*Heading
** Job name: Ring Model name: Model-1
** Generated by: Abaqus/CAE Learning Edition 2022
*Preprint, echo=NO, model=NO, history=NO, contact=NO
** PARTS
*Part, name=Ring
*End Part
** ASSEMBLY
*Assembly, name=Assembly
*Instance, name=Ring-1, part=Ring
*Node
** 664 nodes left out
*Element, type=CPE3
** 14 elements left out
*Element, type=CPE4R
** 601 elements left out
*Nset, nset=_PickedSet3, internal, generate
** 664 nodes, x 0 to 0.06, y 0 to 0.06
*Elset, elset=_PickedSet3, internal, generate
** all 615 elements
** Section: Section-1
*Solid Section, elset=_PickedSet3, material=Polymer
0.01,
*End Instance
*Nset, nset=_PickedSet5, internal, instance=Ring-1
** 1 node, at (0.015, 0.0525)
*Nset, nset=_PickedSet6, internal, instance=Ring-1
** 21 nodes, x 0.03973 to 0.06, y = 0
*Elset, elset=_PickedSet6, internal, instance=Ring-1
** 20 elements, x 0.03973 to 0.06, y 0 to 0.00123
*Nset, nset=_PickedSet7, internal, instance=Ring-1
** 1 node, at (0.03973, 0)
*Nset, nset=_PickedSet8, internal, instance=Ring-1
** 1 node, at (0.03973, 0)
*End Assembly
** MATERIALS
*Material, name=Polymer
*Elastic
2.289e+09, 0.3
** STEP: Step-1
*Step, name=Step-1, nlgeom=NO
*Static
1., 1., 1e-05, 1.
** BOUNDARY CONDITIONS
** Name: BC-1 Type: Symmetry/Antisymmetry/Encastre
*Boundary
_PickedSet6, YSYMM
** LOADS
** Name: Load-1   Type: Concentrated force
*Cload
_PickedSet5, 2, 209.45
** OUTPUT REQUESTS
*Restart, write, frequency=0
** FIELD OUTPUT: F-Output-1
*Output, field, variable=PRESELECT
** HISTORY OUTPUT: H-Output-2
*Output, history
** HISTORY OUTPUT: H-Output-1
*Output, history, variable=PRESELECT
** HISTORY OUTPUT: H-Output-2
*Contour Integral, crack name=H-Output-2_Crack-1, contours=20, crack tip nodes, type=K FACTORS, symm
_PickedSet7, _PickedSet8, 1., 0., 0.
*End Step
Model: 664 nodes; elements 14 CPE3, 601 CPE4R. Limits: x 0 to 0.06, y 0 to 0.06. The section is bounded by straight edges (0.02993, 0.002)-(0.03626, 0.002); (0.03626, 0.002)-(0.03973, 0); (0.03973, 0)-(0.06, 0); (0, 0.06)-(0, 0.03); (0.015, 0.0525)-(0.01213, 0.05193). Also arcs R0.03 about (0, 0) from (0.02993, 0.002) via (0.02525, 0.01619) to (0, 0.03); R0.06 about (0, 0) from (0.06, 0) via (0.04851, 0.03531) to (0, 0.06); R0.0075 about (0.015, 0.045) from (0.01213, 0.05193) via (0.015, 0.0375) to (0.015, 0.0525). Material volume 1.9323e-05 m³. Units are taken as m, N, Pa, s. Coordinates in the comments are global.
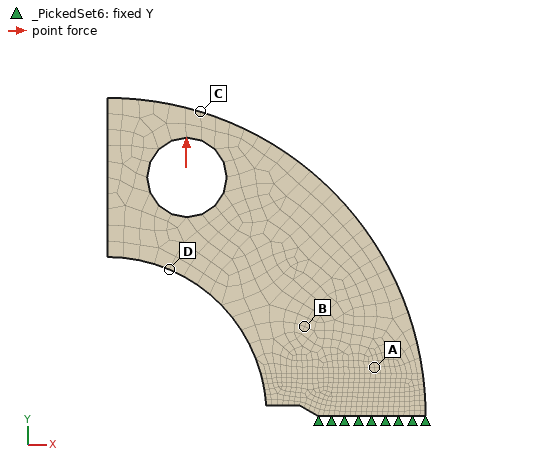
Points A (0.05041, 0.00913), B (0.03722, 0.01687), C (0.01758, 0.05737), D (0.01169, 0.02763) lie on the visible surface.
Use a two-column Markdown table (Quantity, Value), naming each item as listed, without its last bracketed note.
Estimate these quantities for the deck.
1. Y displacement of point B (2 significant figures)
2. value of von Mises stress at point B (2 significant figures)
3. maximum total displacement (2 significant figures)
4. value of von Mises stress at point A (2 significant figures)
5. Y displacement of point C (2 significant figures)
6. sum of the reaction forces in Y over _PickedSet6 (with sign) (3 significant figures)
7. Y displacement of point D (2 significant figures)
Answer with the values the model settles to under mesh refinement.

| Quantity | Value |
|---|---|
| Y displacement of point B | 5.0e-05 m |
| value of von Mises stress at point B | 2.0e+06 Pa |
| maximum total displacement | 4.3e-04 m |
| value of von Mises stress at point A | 2.6e+06 Pa |
| Y displacement of point C | 2.5e-04 m |
| sum of the reaction forces in Y over _PickedSet6 (with sign) | -209 N |
| Y displacement of point D | 2.4e-04 m |
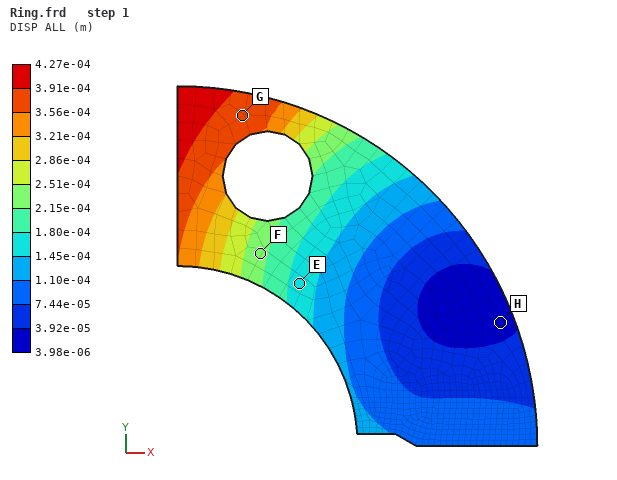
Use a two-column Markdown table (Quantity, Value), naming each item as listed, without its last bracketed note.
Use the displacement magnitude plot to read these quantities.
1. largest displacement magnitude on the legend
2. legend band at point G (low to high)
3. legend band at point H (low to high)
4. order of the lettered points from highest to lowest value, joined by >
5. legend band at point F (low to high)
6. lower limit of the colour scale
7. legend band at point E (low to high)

| Quantity | Value |
|---|---|
| largest displacement magnitude on the legend | 4.27e-04 m |
| legend band at point G | 3.56e-04 to 3.91e-04 m |
| legend band at point H | 3.98e-06 to 3.92e-05 m |
| order of the lettered points from highest to lowest value, joined by > | G > F > E > H |
| legend band at point F | 2.15e-04 to 2.51e-04 m |
| lower limit of the colour scale | 3.98e-06 m |
| legend band at point E | 1.45e-04 to 1.80e-04 m |
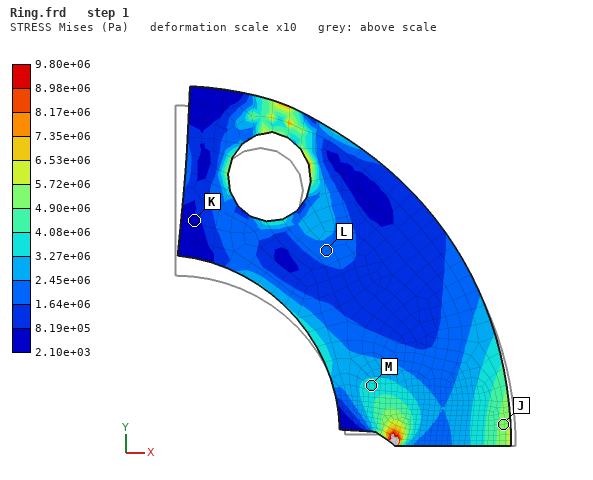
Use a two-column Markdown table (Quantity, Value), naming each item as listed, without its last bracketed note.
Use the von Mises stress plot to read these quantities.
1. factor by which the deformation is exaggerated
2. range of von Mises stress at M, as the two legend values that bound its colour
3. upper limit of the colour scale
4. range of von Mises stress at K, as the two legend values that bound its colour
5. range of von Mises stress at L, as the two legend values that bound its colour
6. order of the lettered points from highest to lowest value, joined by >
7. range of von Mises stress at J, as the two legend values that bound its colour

| Quantity | Value |
|---|---|
| factor by which the deformation is exaggerated | 10 |
| range of von Mises stress at M, as the two legend values that bound its colour | 3.27e+06 to 4.08e+06 Pa |
| upper limit of the colour scale | 9.80e+06 Pa |
| range of von Mises stress at K, as the two legend values that bound its colour | 2.10e+03 to 8.19e+05 Pa |
| range of von Mises stress at L, as the two legend values that bound its colour | 1.64e+06 to 2.45e+06 Pa |
| order of the lettered points from highest to lowest value, joined by > | J > M > L > K |
| range of von Mises stress at J, as the two legend values that bound its colour | 4.90e+06 to 5.72e+06 Pa |
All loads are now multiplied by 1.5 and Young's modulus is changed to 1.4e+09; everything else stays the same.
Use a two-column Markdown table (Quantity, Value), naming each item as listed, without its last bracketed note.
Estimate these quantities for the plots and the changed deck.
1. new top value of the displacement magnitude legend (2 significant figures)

| Quantity | Value |
|---|---|
| new top value of the displacement magnitude legend | 0.0010 m |
